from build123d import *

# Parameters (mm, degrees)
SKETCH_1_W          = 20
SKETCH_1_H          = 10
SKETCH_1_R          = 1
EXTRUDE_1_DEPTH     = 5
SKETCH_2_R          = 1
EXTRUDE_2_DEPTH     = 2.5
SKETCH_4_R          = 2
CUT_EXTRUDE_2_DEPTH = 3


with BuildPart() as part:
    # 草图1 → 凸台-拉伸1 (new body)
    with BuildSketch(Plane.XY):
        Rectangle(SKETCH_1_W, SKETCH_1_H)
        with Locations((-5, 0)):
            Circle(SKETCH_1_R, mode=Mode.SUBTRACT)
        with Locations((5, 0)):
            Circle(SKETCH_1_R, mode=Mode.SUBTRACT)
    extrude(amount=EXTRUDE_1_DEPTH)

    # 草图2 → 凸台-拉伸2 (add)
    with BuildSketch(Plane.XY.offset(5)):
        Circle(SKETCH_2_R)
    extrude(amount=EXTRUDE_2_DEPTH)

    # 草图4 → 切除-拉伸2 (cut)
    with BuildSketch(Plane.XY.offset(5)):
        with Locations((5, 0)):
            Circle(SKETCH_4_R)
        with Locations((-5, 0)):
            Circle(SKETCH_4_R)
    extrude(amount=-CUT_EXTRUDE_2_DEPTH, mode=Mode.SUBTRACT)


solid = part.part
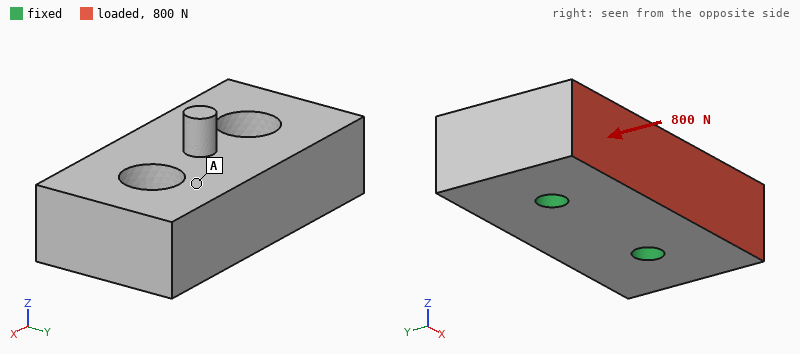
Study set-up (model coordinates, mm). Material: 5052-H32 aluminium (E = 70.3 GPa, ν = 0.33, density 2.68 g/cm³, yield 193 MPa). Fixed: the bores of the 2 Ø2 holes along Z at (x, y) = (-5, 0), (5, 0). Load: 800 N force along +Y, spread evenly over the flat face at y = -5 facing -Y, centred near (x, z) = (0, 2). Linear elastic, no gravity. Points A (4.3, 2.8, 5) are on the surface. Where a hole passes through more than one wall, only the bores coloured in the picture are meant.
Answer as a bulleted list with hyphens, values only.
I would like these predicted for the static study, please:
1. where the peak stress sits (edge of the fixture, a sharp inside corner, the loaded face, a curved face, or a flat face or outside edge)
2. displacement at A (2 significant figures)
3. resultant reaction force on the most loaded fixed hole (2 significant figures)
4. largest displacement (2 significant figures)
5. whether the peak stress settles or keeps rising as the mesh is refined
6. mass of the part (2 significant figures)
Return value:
- edge of the fixture
- 6.5 µm
- 400 N
- 9.5 µm
- keeps rising
- 2.5 g
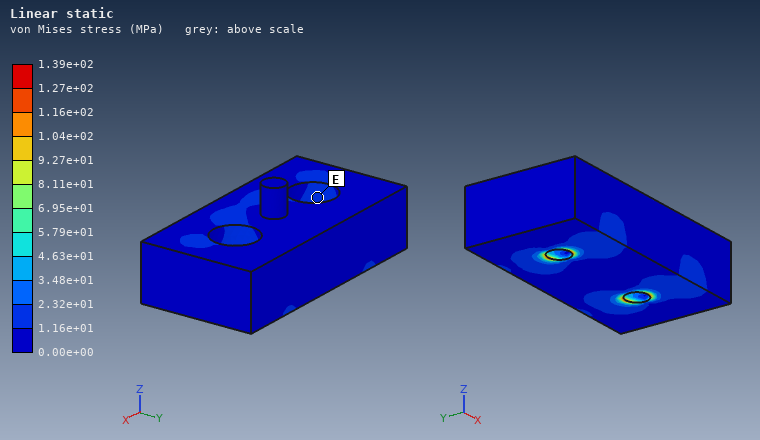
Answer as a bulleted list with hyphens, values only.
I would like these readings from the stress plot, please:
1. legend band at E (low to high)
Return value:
- 1.16e+01 to 2.32e+01 MPa
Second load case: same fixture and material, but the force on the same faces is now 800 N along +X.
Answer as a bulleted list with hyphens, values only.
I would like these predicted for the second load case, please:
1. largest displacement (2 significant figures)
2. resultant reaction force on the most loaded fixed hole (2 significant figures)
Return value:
- 7.4 µm
- 540 N
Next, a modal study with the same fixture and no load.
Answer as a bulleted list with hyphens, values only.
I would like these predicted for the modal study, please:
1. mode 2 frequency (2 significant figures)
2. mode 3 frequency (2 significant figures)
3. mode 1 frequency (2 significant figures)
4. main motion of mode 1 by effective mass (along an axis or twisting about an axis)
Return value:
- 50 kHz
- 50 kHz
- 28 kHz
- along Y
